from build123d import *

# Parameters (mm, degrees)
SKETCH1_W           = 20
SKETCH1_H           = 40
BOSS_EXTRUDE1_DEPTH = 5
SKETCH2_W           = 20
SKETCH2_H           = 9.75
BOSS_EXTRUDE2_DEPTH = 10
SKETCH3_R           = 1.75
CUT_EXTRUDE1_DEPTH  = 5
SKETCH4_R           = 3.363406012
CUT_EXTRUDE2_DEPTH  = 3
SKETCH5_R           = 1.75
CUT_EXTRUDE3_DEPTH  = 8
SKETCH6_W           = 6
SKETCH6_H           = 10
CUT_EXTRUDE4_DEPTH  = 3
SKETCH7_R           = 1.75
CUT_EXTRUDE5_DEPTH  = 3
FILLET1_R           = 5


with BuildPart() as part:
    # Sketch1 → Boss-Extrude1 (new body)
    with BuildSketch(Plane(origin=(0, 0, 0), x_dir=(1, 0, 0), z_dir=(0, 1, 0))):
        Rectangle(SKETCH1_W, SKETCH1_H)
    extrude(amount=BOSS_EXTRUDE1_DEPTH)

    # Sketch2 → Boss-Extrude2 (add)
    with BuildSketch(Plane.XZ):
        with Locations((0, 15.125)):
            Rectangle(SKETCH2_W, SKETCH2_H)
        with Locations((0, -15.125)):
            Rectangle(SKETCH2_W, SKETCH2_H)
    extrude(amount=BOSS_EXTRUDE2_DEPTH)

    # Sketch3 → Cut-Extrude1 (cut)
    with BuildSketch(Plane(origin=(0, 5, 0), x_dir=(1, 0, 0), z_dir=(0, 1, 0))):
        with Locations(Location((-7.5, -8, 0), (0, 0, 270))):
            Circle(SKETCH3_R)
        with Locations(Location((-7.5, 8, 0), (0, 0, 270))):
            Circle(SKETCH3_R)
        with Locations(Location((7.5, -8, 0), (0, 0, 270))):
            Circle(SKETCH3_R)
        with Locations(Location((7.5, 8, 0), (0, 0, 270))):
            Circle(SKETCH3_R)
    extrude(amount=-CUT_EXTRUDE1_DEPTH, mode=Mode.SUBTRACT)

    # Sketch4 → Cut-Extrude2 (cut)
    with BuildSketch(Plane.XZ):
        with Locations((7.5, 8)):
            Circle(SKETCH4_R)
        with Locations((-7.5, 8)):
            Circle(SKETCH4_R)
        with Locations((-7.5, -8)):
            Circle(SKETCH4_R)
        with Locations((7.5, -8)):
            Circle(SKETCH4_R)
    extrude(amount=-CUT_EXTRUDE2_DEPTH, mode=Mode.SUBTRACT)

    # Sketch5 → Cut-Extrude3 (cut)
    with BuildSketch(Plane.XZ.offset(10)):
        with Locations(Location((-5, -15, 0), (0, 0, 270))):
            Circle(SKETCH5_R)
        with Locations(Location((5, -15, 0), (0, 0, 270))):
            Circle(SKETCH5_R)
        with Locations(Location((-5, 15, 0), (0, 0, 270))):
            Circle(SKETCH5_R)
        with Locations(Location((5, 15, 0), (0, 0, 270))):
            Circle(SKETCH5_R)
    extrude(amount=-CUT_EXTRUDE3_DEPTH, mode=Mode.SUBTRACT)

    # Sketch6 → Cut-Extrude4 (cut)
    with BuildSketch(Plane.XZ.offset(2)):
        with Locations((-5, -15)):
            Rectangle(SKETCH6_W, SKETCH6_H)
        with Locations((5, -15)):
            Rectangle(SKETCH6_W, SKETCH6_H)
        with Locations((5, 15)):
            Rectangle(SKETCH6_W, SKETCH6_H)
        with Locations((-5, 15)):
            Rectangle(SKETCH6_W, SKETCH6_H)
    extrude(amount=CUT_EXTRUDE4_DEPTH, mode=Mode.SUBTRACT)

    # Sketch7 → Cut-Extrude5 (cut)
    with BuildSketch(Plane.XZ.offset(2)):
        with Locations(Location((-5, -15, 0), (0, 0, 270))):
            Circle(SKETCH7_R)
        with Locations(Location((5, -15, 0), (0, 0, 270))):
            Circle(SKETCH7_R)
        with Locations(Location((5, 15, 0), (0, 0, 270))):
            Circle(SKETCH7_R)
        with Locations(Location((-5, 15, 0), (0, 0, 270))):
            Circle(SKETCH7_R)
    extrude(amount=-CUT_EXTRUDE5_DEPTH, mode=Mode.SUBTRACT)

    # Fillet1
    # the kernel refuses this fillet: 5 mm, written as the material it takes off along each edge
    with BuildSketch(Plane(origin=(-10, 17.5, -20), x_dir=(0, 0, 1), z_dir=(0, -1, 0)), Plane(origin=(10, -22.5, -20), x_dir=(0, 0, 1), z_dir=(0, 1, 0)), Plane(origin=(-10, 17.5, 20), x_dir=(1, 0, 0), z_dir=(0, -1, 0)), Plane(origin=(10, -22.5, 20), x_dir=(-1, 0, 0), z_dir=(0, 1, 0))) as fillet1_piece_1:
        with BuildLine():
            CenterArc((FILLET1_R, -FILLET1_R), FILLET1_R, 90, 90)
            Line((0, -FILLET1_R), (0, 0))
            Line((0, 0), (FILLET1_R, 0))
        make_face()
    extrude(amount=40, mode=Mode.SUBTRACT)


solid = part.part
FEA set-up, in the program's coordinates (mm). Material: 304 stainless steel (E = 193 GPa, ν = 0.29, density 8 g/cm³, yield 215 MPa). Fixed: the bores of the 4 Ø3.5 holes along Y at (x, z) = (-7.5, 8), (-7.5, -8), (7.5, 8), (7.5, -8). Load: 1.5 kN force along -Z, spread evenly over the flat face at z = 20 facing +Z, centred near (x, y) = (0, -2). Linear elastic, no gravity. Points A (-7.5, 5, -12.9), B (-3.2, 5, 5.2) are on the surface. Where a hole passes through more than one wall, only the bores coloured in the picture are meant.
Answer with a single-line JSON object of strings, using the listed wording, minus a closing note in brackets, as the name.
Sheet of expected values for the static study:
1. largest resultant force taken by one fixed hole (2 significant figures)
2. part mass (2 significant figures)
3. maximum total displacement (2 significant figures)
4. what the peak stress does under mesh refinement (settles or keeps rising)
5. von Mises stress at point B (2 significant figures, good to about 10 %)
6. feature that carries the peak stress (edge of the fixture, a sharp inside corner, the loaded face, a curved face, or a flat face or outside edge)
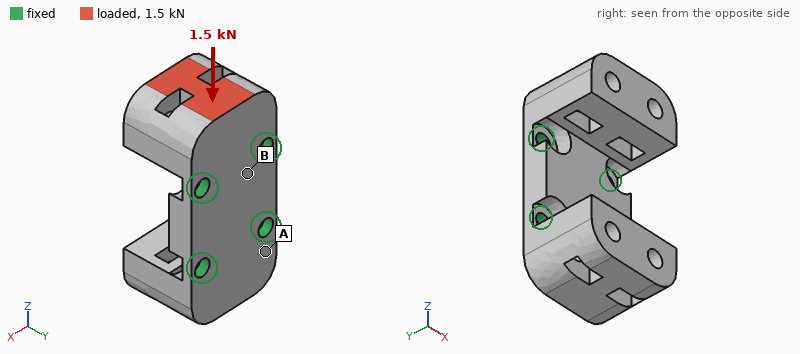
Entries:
{"largest resultant force taken by one fixed hole": "580 N", "part mass": "49 g", "maximum total displacement": "40 µm", "what the peak stress does under mesh refinement": "keeps rising", "von Mises stress at point B": "33 MPa", "feature that carries the peak stress": "edge of the fixture"}
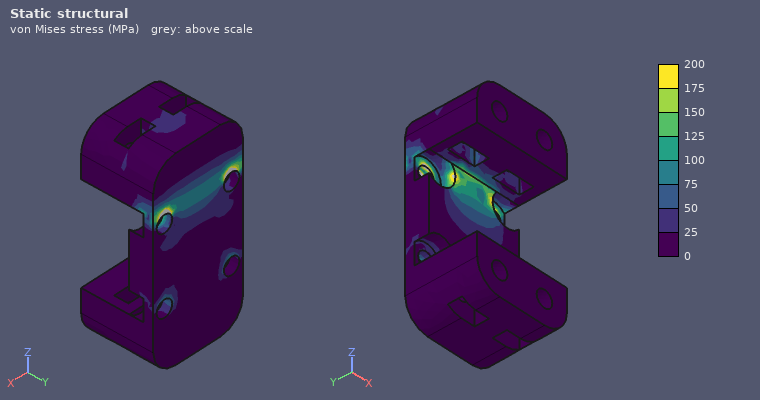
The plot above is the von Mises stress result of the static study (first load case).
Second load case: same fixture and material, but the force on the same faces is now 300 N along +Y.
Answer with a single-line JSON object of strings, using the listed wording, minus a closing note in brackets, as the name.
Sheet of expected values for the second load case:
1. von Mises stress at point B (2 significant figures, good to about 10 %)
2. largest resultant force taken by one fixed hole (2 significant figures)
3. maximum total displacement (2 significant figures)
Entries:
{"von Mises stress at point B": "14 MPa", "largest resultant force taken by one fixed hole": "280 N", "maximum total displacement": "14 µm"}
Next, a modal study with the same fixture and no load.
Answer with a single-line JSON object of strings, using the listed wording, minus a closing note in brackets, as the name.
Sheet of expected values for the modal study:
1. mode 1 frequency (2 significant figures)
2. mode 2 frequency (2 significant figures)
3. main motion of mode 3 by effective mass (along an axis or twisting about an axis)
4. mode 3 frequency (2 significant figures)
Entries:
{"mode 1 frequency": "7700 Hz", "mode 2 frequency": "7900 Hz", "main motion of mode 3 by effective mass": "along X", "mode 3 frequency": "16 kHz"}
